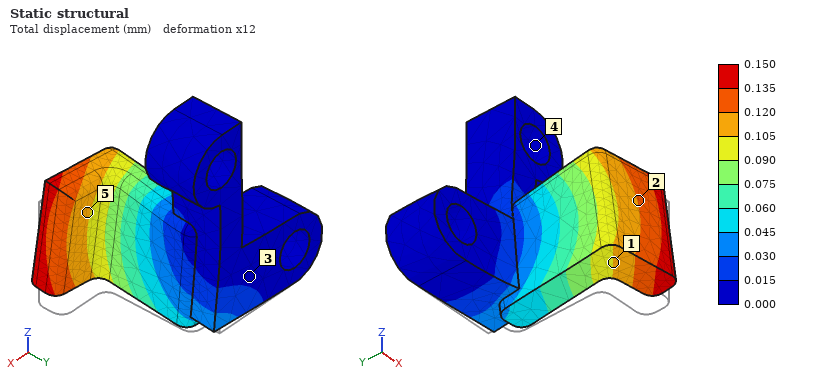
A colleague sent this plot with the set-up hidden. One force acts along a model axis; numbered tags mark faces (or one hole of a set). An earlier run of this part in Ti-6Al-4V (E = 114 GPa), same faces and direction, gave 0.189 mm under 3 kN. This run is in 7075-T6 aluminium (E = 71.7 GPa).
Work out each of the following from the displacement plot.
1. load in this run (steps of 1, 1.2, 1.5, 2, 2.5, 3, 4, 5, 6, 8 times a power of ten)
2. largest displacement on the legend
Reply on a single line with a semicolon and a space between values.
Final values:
1.5 kN; 0.150 mm
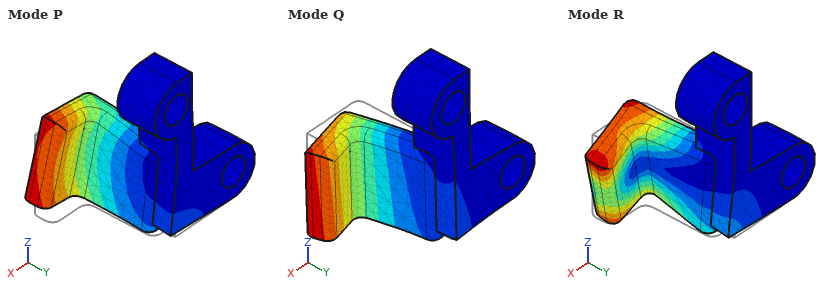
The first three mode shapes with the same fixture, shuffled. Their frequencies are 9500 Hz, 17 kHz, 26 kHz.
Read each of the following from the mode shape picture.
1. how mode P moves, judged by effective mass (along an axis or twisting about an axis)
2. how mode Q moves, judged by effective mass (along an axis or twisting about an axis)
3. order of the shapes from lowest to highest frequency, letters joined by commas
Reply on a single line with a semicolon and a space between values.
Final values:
along Z; along X; Q, P, R
